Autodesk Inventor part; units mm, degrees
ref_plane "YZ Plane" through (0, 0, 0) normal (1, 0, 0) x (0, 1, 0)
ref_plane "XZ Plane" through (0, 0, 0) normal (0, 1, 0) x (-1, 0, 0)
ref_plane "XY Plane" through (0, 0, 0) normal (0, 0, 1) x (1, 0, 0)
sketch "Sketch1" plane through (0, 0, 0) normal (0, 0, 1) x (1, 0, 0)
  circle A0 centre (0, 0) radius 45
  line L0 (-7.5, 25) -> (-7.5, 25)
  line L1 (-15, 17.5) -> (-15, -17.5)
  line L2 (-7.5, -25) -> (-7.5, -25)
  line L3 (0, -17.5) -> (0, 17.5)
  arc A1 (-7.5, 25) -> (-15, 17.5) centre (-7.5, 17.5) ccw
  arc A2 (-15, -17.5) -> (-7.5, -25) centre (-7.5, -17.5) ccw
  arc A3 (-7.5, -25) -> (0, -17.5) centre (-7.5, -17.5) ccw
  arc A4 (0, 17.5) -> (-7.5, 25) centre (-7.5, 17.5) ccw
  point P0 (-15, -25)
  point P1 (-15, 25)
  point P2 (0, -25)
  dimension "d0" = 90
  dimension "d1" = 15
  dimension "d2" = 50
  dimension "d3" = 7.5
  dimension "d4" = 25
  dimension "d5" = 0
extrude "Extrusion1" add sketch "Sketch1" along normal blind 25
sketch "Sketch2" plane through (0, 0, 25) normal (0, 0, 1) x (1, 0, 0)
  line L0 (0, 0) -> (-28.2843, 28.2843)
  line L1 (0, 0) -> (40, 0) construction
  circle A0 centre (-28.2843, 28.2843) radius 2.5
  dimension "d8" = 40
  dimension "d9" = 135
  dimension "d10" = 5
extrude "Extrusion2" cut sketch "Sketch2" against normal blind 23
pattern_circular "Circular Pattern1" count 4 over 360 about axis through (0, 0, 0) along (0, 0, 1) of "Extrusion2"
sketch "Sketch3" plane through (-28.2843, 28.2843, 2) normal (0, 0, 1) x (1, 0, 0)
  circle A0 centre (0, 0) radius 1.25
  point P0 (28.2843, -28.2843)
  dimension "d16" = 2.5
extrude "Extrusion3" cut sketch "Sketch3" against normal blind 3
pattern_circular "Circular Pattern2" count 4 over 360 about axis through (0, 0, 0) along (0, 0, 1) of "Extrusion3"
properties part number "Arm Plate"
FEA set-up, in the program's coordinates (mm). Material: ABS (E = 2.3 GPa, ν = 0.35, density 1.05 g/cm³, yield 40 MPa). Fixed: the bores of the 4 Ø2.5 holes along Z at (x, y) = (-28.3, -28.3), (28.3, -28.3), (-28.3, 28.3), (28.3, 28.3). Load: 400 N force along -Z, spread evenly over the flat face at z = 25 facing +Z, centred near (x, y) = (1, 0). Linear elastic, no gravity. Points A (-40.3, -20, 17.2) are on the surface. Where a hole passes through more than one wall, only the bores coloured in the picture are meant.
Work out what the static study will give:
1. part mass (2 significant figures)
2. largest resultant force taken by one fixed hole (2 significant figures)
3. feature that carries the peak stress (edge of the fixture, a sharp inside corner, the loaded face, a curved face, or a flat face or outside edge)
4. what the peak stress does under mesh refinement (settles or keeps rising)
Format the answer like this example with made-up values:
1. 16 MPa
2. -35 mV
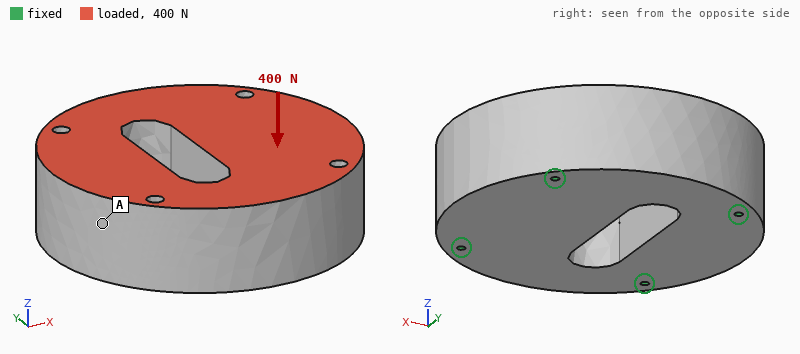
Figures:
1. 150 g
2. 110 N
3. edge of the fixture
4. keeps rising
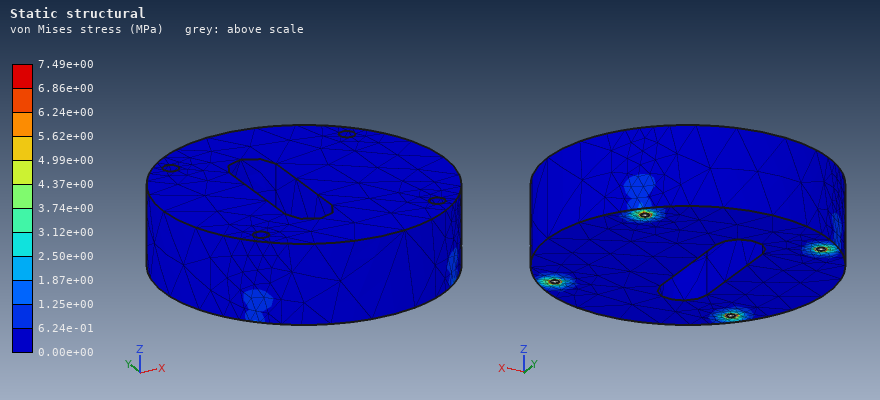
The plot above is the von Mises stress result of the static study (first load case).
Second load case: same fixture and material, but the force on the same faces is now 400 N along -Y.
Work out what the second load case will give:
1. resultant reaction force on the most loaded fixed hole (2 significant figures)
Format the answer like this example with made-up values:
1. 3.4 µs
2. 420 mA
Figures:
1. 140 N
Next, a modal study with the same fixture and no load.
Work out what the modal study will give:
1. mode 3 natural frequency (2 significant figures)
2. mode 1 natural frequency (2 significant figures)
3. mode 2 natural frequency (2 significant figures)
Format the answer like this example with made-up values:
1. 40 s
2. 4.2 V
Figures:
1. 1900 Hz
2. 1800 Hz
3. 1900 Hz
